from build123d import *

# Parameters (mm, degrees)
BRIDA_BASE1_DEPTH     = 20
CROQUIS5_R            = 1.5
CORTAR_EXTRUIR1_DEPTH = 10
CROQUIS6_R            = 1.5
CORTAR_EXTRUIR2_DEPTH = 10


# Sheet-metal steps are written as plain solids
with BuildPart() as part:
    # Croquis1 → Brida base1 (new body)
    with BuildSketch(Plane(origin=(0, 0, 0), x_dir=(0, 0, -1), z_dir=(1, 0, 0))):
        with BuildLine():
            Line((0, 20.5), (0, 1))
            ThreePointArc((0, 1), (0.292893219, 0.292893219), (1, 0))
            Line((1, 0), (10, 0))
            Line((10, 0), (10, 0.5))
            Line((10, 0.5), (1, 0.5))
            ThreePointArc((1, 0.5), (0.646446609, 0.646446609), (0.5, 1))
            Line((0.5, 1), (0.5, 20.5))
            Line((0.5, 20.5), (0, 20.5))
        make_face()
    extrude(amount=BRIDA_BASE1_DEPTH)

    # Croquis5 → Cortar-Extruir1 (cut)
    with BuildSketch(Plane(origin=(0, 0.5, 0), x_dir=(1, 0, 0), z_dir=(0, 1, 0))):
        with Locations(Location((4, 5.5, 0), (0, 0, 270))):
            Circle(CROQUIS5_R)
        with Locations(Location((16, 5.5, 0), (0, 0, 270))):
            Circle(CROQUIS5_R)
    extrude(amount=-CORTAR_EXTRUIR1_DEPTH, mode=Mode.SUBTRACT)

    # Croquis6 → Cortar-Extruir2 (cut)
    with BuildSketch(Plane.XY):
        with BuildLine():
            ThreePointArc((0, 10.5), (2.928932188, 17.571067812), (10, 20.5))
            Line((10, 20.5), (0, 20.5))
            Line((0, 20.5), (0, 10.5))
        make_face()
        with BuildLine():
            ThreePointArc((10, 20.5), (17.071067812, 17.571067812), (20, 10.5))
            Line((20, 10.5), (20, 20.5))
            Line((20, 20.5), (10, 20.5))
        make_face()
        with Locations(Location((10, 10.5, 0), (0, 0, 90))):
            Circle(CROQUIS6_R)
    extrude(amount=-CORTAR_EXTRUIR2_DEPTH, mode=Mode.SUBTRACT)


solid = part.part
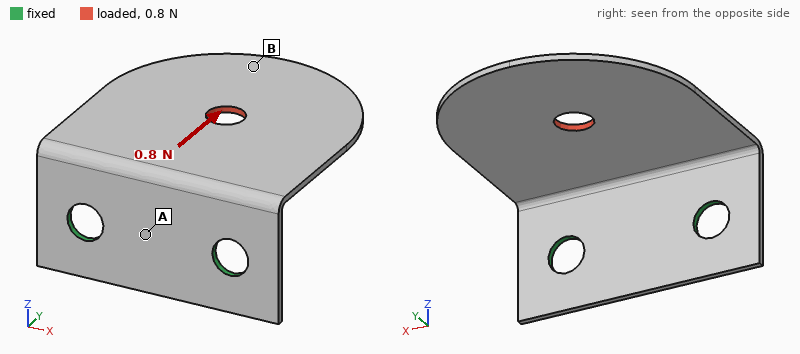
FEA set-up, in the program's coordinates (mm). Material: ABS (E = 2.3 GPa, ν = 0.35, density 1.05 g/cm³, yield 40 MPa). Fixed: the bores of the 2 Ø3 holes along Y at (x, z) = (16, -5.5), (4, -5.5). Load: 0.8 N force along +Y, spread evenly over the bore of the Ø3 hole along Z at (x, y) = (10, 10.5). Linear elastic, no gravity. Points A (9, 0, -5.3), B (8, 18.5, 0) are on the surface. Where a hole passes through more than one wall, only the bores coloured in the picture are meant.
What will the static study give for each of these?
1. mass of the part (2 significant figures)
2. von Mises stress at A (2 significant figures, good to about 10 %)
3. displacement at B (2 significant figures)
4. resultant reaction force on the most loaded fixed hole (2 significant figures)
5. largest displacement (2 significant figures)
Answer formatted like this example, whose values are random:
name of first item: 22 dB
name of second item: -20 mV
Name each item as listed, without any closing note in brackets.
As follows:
mass of the part: 0.28 g
von Mises stress at A: 0.92 MPa
displacement at B: 0.27 mm
resultant reaction force on the most loaded fixed hole: 0.40 N
largest displacement: 0.29 mm
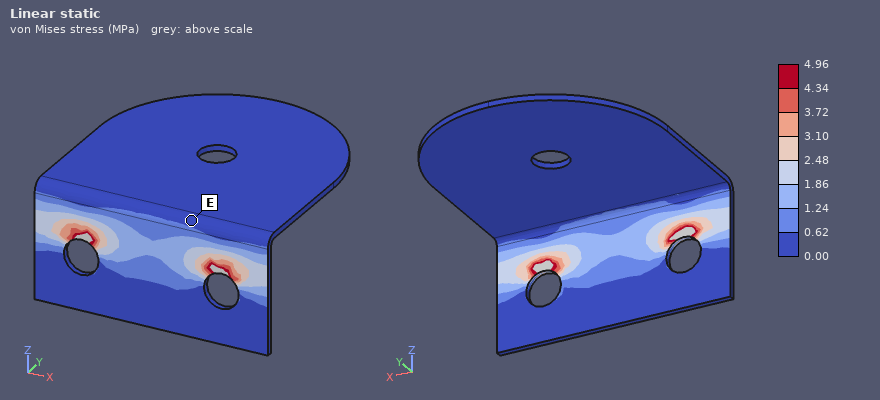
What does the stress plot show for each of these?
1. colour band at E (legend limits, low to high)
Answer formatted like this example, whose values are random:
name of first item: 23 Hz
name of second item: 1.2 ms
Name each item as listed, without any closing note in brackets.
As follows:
colour band at E: 0.00 to 0.62 MPa
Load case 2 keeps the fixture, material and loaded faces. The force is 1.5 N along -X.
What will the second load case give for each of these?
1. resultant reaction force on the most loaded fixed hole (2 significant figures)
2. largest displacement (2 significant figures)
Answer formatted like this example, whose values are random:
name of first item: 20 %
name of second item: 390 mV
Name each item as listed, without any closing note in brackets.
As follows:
resultant reaction force on the most loaded fixed hole: 1.5 N
largest displacement: 0.29 mm
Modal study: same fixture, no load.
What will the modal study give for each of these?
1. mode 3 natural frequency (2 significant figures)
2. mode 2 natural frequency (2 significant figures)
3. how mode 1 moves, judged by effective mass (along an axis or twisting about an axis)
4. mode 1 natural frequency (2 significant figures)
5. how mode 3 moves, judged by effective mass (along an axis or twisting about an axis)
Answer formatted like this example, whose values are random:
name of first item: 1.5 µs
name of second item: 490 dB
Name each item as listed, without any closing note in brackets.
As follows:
mode 3 natural frequency: 1200 Hz
mode 2 natural frequency: 770 Hz
how mode 1 moves, judged by effective mass: along Z
mode 1 natural frequency: 270 Hz
how mode 3 moves, judged by effective mass: along X
